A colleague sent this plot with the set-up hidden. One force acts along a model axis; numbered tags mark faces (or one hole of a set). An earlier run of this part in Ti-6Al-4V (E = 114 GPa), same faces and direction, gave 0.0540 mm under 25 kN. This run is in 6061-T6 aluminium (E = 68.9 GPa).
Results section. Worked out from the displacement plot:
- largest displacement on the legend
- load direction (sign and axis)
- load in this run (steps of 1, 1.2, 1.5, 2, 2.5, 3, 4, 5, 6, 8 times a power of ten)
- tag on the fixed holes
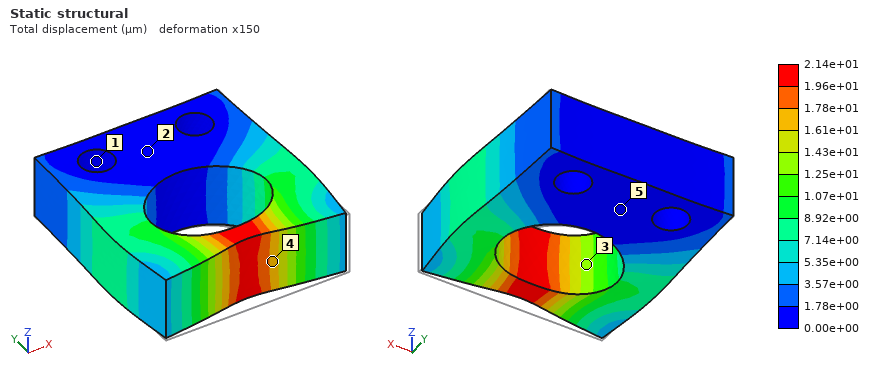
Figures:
2.14e+01 µm
+Y
6 kN
1
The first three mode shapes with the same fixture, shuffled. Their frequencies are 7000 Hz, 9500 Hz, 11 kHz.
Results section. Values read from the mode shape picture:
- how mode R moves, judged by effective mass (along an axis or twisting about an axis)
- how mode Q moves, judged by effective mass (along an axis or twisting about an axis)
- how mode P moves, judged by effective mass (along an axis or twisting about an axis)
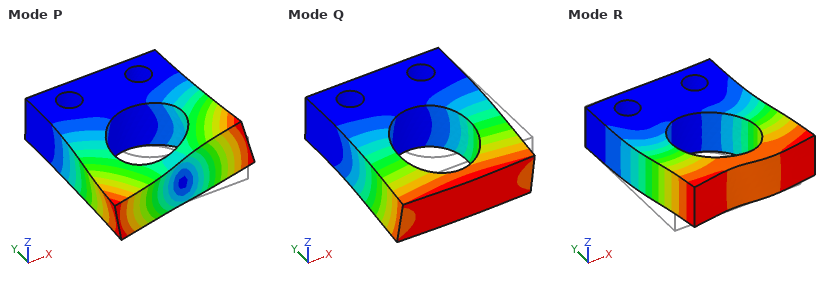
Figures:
along X
along Z
twisting about Y
